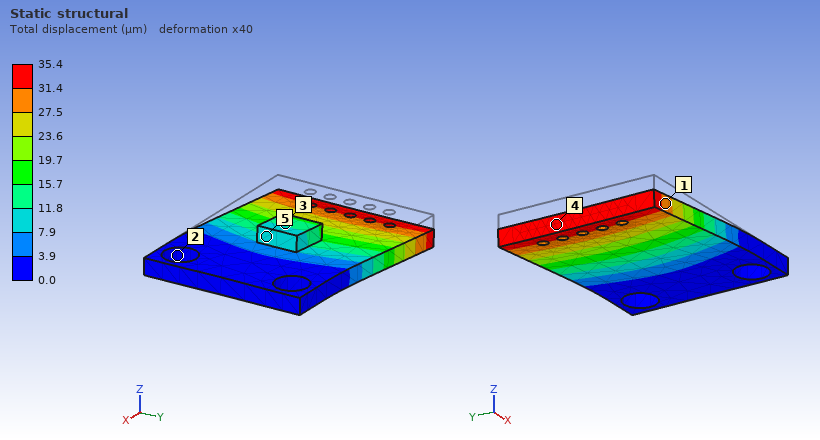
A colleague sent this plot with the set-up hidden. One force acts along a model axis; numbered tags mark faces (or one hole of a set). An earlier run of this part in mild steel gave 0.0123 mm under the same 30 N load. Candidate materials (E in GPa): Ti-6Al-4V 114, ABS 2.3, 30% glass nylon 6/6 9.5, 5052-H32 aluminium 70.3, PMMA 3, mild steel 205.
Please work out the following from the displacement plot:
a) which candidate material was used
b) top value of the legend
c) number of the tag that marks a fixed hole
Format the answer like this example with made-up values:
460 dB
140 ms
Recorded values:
5052-H32 aluminium
35.4 µm
2
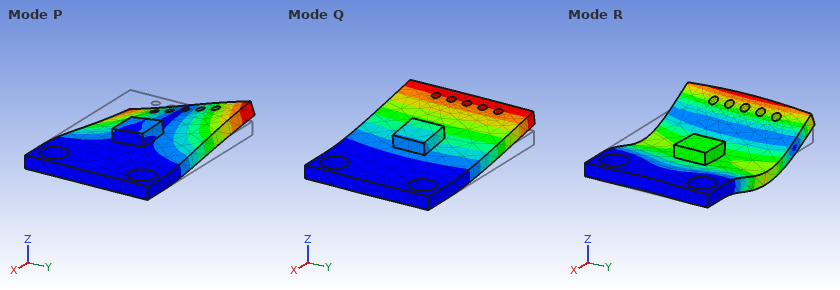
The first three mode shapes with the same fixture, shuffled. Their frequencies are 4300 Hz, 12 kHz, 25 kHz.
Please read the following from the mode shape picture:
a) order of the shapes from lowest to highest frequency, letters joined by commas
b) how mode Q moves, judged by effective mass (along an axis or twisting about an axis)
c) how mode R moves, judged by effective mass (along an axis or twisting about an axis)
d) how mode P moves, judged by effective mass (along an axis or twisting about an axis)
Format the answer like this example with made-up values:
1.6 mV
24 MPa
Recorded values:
Q, P, R
along Z
along Z
twisting about X
